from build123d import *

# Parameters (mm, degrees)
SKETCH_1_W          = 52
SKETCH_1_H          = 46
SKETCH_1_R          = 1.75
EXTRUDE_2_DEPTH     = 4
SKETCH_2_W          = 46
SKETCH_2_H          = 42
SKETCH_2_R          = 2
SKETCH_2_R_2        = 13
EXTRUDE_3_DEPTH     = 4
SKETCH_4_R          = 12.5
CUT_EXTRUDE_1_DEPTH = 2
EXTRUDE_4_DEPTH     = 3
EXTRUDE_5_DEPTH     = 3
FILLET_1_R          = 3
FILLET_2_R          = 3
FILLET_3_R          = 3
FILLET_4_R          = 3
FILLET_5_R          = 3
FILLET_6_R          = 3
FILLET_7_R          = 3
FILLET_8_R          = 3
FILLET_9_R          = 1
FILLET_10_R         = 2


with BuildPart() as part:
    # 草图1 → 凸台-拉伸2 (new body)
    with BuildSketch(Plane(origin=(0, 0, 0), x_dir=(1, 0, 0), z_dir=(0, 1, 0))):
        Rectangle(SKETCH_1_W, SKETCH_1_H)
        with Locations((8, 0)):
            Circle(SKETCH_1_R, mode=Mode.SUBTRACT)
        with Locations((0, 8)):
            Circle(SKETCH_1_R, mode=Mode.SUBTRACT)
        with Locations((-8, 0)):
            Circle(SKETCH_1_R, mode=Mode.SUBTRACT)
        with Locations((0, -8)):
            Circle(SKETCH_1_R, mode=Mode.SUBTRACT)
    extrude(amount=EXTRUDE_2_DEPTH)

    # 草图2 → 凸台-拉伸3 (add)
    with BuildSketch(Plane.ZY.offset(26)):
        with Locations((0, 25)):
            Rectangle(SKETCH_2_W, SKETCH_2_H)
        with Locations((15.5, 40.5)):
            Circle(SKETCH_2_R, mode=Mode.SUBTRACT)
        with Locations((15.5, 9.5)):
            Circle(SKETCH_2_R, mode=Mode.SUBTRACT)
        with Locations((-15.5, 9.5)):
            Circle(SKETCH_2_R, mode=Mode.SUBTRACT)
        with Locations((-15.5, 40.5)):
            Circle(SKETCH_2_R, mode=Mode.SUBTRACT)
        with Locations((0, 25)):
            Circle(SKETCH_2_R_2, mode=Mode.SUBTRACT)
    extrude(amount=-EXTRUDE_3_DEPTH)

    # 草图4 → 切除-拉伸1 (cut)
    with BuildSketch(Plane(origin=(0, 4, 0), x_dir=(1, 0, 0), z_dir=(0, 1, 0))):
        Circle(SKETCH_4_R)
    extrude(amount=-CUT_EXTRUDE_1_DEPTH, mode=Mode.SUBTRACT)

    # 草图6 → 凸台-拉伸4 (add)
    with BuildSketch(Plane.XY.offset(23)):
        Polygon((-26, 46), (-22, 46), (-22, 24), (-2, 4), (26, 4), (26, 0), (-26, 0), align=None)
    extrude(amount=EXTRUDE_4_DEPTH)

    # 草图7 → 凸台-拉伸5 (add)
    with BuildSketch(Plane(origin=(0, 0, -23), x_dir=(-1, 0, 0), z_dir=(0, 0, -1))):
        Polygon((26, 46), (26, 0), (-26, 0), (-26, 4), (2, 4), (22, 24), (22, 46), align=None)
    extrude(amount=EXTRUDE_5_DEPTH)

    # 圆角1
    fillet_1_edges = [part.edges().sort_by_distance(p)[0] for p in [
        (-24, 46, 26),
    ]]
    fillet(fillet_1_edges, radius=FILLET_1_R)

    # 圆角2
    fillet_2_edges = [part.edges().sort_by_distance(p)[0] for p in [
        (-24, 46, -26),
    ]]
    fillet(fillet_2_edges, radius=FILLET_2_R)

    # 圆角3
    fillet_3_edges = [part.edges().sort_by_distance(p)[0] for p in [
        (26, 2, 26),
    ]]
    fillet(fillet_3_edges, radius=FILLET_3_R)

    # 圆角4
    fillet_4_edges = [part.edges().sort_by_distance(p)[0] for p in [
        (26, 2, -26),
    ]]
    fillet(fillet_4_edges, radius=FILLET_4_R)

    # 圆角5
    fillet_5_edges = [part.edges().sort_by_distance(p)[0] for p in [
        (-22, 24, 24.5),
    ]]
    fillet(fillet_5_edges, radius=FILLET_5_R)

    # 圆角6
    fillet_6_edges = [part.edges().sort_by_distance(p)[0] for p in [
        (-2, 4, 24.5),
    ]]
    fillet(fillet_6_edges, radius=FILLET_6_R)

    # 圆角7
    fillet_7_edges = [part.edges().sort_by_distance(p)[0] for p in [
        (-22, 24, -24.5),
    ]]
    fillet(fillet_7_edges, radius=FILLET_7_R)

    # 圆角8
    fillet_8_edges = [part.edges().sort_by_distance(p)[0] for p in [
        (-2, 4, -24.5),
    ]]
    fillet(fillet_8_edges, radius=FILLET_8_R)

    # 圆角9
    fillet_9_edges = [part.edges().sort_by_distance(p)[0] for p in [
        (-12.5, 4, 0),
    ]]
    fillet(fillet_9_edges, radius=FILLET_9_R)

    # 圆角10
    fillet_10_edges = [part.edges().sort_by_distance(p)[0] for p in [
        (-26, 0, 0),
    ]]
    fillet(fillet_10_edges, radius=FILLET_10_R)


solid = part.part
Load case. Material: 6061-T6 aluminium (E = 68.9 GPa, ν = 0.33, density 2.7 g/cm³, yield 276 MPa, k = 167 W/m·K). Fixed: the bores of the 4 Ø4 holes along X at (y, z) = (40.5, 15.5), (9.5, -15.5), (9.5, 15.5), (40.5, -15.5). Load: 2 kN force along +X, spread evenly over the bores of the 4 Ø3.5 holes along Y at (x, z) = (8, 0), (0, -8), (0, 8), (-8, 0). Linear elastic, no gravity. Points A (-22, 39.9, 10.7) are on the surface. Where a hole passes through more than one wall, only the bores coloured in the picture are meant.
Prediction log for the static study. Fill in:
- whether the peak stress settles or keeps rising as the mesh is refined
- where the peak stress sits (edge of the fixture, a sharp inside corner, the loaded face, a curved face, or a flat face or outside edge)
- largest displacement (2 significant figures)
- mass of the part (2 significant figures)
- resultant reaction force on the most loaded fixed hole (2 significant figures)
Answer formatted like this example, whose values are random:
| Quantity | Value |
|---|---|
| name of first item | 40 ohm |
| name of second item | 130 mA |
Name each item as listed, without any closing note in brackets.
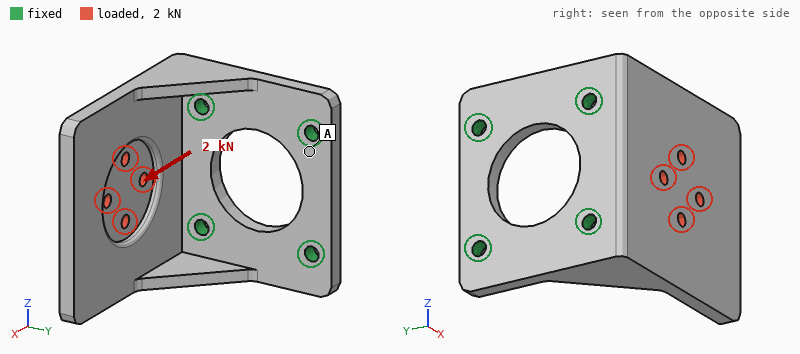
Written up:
| Quantity | Value |
|---|---|
| whether the peak stress settles or keeps rising as the mesh is refined | keeps rising |
| where the peak stress sits | edge of the fixture |
| largest displacement | 0.15 mm |
| mass of the part | 47 g |
| resultant reaction force on the most loaded fixed hole | 1.1 kN |
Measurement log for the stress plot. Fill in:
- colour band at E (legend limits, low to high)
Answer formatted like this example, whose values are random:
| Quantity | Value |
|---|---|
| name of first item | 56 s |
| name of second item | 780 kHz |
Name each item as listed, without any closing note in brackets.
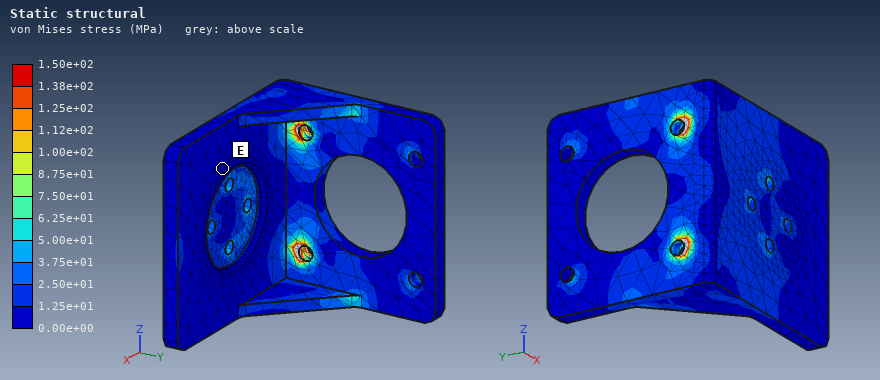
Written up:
| Quantity | Value |
|---|---|
| colour band at E | 0.00e+00 to 1.25e+01 MPa |
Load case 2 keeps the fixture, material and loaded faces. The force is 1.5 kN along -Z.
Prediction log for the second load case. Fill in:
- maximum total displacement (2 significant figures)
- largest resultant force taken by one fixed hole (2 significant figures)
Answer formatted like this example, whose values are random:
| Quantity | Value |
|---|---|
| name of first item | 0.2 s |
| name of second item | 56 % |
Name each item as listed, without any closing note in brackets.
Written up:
| Quantity | Value |
|---|---|
| maximum total displacement | 81 µm |
| largest resultant force taken by one fixed hole | 1.3 kN |
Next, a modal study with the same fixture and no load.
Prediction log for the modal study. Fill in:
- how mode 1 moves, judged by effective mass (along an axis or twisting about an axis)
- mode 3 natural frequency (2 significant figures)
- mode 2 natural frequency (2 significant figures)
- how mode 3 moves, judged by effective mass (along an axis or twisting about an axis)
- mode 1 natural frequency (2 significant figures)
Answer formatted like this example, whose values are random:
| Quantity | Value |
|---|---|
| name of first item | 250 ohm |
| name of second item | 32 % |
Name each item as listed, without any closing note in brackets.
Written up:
| Quantity | Value |
|---|---|
| how mode 1 moves, judged by effective mass | along Y |
| mode 3 natural frequency | 5800 Hz |
| mode 2 natural frequency | 3500 Hz |
| how mode 3 moves, judged by effective mass | along Z |
| mode 1 natural frequency | 1600 Hz |
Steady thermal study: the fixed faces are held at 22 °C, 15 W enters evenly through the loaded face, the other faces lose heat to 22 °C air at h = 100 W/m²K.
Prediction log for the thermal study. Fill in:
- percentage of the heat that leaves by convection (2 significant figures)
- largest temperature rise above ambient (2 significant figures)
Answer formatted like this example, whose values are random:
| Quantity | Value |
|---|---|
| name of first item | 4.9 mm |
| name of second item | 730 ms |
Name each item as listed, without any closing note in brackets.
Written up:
| Quantity | Value |
|---|---|
| percentage of the heat that leaves by convection | 32 % |
| largest temperature rise above ambient | 14 K |
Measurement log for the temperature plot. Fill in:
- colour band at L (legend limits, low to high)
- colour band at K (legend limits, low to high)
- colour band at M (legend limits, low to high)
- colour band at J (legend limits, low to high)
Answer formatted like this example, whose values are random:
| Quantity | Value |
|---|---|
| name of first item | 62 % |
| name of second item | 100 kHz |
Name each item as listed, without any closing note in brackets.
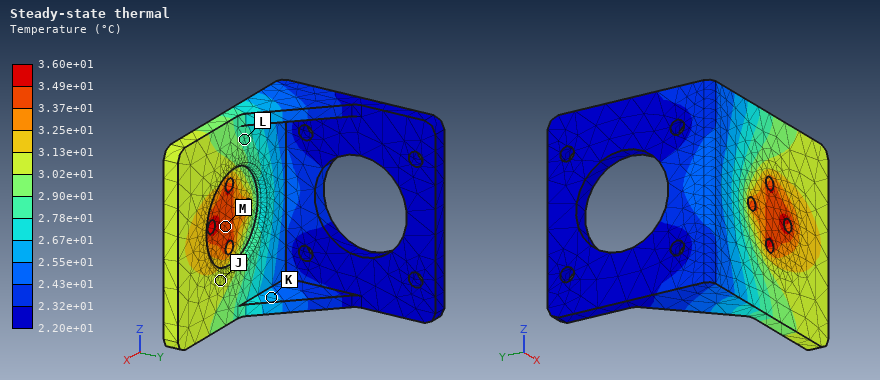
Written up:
| Quantity | Value |
|---|---|
| colour band at L | 2.78e+01 to 2.90e+01 °C |
| colour band at K | 2.55e+01 to 2.67e+01 °C |
| colour band at M | 3.37e+01 to 3.49e+01 °C |
| colour band at J | 3.02e+01 to 3.13e+01 °C |
